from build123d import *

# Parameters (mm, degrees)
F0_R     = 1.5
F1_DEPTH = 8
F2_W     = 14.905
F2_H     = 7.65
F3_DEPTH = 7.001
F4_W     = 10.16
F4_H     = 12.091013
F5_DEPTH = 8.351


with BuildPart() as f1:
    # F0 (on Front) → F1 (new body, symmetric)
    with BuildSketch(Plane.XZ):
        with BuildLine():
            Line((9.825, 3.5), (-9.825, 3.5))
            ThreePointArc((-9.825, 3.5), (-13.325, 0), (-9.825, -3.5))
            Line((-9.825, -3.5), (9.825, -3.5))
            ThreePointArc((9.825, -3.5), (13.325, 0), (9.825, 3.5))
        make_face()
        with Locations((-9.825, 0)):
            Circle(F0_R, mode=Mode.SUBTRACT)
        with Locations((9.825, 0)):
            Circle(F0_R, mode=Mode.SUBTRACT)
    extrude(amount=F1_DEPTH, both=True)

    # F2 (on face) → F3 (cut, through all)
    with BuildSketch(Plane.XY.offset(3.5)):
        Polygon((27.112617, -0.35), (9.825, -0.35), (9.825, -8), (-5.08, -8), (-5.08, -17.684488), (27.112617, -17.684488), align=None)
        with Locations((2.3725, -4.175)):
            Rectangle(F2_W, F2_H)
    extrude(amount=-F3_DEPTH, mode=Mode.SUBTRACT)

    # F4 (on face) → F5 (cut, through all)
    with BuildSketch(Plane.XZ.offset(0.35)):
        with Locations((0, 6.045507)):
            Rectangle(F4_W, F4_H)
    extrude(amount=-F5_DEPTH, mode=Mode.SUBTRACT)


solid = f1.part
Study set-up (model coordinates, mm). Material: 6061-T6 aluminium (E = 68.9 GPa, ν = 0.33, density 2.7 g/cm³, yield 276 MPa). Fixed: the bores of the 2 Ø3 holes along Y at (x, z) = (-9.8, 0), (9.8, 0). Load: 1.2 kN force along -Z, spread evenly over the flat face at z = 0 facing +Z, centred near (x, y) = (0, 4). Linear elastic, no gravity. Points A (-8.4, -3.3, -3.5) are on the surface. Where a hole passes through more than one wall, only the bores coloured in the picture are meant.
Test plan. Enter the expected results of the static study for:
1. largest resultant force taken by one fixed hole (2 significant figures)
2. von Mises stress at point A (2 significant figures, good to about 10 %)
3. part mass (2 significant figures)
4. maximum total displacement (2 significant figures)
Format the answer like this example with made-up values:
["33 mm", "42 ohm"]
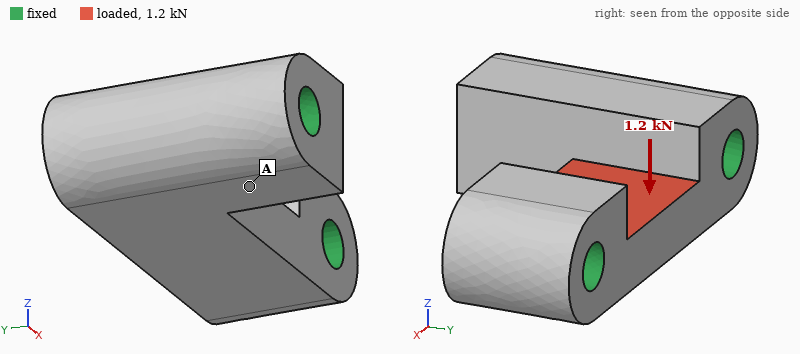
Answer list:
["670 N", "12 MPa", "3.8 g", "12 µm"]
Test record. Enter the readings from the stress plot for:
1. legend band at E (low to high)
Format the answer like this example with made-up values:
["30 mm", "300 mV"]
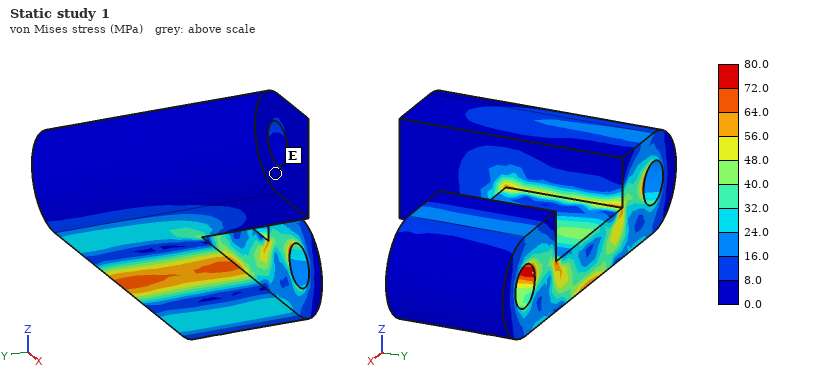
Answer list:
["0.0 to 8.0 MPa"]
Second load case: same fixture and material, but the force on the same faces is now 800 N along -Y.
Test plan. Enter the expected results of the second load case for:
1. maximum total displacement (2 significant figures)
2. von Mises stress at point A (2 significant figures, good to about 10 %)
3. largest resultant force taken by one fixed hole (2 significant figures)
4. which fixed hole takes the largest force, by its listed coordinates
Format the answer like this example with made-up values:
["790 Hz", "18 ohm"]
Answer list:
["7.2 µm", "8.3 MPa", "430 N", "(-9.8, 0)"]
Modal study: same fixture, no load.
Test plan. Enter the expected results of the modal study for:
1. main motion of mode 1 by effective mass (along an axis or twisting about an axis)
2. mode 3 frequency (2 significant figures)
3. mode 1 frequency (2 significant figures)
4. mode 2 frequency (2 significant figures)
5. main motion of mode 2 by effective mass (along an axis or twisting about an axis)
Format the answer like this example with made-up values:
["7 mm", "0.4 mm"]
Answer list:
["along Z", "89 kHz", "62 kHz", "80 kHz", "along Y"]
